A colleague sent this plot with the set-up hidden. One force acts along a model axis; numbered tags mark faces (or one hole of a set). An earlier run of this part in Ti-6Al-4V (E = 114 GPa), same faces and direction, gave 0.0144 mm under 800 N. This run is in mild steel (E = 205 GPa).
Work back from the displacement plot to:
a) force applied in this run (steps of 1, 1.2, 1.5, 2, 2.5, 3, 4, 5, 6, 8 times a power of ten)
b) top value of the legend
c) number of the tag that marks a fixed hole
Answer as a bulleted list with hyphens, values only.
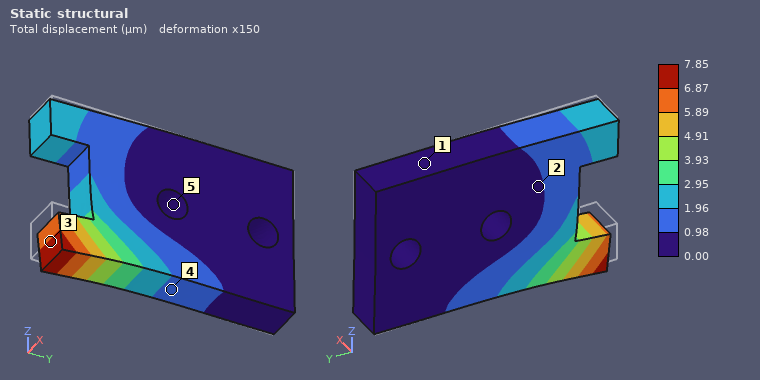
- 800 N
- 7.85 µm
- 5
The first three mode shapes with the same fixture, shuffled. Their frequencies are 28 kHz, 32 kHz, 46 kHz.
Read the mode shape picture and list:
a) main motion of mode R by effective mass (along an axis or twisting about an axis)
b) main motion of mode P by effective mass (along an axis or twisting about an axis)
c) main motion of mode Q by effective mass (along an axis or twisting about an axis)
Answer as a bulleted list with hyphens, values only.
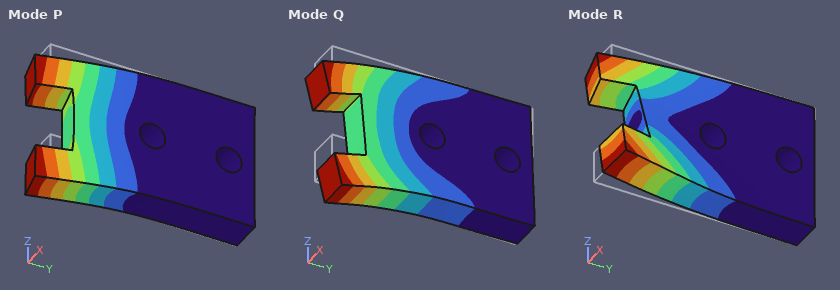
- twisting about Y
- along X
- along Z
